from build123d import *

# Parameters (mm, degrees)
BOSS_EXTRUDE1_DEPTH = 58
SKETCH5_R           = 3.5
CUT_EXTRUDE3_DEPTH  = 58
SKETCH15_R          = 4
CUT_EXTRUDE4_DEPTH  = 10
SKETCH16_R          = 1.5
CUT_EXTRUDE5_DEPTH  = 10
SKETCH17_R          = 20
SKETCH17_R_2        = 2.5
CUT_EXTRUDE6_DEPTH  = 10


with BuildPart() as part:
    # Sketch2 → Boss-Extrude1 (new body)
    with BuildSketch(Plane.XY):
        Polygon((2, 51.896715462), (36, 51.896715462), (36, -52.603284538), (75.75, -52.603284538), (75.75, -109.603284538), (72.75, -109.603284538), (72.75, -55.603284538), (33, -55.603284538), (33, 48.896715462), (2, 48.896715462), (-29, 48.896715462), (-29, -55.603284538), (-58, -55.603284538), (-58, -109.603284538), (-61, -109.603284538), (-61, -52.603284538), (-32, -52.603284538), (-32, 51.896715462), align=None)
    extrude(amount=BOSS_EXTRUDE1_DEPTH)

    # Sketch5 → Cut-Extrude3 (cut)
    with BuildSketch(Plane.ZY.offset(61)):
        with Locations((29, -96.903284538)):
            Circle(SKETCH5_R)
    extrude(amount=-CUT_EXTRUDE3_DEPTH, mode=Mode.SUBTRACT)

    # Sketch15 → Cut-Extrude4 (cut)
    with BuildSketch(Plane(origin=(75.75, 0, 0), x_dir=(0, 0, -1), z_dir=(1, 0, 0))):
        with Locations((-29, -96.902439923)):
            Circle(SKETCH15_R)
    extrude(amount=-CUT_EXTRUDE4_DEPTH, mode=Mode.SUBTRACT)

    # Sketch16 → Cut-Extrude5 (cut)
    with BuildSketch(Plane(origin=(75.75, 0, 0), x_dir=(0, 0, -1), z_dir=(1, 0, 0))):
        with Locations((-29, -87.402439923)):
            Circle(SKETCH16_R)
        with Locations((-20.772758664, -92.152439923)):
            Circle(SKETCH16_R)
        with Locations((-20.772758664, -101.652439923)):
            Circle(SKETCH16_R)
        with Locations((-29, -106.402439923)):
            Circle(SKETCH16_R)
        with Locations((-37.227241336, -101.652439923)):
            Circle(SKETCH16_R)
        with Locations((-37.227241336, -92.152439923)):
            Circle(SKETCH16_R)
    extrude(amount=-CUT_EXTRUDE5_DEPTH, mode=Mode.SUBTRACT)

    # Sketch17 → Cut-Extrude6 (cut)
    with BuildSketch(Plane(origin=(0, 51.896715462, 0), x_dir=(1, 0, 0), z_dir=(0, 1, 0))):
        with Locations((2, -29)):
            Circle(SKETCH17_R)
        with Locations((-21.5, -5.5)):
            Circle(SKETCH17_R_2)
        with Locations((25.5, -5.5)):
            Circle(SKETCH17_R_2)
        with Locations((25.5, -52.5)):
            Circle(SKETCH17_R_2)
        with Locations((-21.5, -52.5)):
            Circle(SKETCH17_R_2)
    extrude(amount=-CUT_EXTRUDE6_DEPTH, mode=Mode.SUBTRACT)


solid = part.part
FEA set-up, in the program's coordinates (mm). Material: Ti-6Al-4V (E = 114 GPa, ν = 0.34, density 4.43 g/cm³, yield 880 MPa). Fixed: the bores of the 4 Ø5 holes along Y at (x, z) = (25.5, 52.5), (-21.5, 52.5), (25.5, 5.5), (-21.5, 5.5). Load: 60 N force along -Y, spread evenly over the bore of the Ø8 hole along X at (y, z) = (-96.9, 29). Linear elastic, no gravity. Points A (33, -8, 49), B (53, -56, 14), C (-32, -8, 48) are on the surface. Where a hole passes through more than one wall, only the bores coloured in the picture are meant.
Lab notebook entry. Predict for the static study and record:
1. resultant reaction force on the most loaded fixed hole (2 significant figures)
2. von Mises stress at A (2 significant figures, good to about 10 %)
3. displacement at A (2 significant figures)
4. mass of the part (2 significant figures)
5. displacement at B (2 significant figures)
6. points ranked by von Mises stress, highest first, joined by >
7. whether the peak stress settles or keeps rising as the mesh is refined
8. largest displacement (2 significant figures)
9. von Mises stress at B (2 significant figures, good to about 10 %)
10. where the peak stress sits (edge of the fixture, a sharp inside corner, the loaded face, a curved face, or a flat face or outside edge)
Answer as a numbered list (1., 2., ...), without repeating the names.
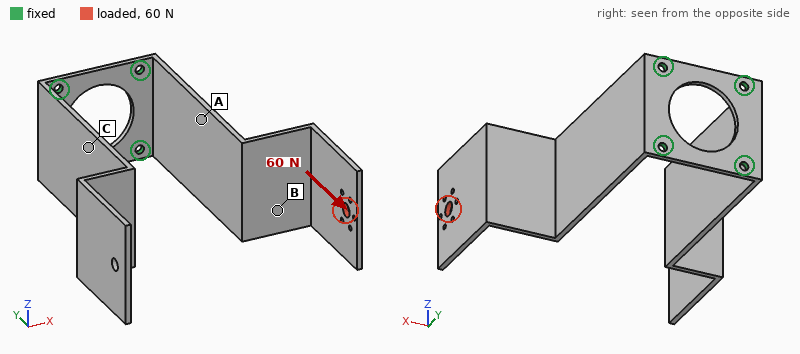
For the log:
1. 33 N
2. 27 MPa
3. 0.35 mm
4. 330 g
5. 1.1 mm
6. A > B > C
7. keeps rising
8. 2.3 mm
9. 13 MPa
10. edge of the fixture
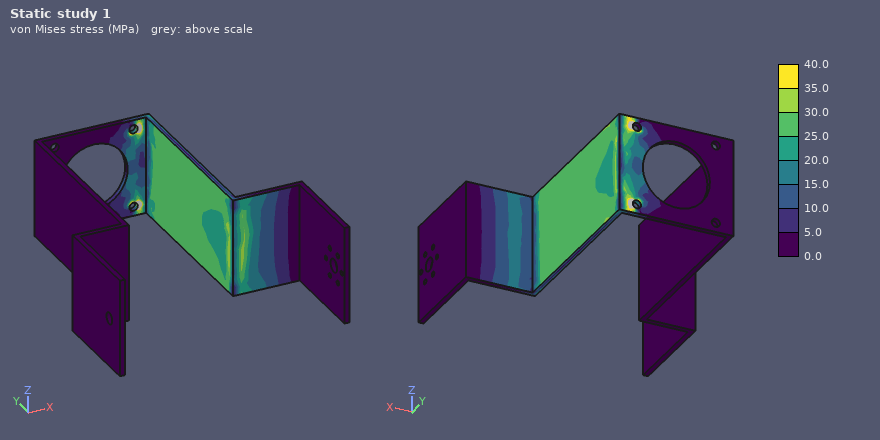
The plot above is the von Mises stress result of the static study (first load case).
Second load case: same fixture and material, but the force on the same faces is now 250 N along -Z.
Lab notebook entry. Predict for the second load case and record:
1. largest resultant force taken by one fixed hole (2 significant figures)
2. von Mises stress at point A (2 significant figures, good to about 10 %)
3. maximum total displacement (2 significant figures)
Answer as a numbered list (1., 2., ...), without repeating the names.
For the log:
1. 840 N
2. 93 MPa
3. 2.2 mm
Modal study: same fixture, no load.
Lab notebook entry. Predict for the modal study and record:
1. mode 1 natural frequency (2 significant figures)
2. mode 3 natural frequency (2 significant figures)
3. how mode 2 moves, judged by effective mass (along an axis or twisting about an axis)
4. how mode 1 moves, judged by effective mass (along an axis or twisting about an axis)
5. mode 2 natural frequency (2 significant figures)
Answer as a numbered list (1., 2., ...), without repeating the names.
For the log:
1. 74 Hz
2. 240 Hz
3. along X
4. along X
5. 78 Hz
